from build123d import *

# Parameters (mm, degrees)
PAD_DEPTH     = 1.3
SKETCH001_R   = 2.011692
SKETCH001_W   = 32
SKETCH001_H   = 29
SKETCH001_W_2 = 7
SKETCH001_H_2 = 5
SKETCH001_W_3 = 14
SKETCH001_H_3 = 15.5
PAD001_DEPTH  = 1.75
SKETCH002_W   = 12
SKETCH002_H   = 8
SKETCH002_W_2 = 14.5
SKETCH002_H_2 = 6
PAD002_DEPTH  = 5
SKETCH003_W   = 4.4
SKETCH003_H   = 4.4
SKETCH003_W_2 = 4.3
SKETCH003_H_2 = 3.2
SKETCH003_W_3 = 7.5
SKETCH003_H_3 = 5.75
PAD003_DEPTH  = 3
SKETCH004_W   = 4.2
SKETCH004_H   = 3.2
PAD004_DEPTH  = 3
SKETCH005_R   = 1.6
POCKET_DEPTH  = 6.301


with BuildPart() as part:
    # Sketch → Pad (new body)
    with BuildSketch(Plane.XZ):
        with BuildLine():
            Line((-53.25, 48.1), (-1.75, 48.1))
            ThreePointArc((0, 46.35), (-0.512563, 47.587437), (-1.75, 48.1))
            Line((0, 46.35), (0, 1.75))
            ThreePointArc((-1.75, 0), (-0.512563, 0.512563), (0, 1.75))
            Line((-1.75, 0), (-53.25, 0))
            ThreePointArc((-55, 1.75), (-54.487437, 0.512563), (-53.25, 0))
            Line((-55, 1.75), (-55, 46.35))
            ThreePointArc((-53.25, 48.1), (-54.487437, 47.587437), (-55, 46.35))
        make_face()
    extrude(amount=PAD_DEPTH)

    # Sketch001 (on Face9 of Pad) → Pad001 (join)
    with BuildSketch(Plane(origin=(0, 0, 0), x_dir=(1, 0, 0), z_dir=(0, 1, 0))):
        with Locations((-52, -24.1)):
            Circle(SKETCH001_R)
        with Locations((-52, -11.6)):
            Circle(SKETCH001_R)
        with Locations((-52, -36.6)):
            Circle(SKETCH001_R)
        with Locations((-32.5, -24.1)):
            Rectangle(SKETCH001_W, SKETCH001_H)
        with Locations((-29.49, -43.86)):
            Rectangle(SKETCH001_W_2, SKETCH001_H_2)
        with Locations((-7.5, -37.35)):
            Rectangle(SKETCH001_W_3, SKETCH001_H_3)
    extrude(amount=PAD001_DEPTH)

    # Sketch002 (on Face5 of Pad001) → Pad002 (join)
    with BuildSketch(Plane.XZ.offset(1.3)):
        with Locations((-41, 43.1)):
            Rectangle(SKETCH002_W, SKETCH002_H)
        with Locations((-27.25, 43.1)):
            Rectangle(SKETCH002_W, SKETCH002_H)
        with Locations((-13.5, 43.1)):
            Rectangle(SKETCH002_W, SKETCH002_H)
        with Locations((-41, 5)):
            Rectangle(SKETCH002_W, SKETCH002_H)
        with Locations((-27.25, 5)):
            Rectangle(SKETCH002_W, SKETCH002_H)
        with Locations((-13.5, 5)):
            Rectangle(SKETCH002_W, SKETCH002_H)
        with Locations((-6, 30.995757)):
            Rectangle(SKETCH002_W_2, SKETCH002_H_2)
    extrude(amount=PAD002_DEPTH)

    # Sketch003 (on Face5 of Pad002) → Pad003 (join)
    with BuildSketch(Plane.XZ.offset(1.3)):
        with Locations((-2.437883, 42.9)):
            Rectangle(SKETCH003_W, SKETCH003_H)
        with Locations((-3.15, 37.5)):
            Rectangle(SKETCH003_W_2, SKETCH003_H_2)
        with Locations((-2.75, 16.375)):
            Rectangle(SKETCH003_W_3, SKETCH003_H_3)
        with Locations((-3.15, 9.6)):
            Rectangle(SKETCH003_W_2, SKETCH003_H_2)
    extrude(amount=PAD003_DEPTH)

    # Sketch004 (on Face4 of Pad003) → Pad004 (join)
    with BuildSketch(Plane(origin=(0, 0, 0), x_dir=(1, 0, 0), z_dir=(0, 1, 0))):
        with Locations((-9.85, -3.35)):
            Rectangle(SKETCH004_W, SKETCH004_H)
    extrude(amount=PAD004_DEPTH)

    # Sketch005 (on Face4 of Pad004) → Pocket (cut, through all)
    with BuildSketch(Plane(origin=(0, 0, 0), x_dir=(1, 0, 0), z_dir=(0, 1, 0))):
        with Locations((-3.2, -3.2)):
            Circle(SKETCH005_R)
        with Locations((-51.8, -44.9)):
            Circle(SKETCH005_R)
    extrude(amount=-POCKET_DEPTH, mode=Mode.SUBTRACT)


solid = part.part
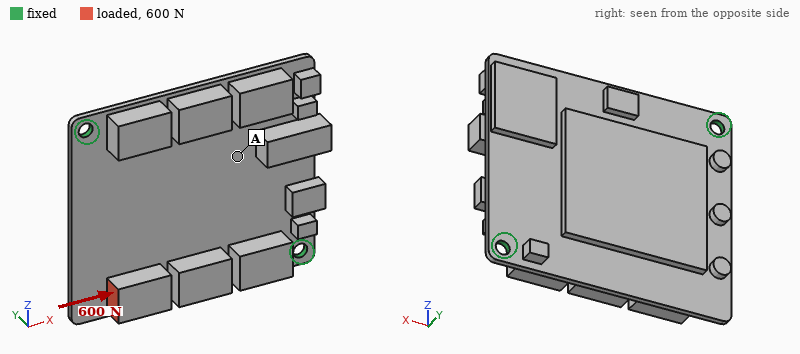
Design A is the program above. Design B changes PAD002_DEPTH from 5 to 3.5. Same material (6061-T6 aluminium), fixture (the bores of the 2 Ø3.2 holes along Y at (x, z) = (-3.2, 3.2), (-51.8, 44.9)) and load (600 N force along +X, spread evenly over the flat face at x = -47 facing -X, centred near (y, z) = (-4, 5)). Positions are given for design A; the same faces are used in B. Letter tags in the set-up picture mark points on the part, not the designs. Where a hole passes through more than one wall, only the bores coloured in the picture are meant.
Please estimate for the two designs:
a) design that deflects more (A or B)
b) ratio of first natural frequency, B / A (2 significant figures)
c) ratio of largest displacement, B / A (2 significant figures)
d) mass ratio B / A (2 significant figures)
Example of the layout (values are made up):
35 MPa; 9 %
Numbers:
A; 1.1; 0.79; 0.89
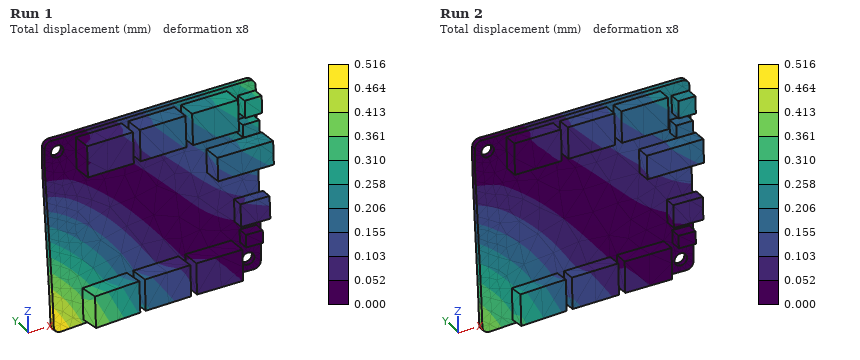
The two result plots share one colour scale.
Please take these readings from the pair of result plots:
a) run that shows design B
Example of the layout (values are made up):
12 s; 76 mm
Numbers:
Run 2
